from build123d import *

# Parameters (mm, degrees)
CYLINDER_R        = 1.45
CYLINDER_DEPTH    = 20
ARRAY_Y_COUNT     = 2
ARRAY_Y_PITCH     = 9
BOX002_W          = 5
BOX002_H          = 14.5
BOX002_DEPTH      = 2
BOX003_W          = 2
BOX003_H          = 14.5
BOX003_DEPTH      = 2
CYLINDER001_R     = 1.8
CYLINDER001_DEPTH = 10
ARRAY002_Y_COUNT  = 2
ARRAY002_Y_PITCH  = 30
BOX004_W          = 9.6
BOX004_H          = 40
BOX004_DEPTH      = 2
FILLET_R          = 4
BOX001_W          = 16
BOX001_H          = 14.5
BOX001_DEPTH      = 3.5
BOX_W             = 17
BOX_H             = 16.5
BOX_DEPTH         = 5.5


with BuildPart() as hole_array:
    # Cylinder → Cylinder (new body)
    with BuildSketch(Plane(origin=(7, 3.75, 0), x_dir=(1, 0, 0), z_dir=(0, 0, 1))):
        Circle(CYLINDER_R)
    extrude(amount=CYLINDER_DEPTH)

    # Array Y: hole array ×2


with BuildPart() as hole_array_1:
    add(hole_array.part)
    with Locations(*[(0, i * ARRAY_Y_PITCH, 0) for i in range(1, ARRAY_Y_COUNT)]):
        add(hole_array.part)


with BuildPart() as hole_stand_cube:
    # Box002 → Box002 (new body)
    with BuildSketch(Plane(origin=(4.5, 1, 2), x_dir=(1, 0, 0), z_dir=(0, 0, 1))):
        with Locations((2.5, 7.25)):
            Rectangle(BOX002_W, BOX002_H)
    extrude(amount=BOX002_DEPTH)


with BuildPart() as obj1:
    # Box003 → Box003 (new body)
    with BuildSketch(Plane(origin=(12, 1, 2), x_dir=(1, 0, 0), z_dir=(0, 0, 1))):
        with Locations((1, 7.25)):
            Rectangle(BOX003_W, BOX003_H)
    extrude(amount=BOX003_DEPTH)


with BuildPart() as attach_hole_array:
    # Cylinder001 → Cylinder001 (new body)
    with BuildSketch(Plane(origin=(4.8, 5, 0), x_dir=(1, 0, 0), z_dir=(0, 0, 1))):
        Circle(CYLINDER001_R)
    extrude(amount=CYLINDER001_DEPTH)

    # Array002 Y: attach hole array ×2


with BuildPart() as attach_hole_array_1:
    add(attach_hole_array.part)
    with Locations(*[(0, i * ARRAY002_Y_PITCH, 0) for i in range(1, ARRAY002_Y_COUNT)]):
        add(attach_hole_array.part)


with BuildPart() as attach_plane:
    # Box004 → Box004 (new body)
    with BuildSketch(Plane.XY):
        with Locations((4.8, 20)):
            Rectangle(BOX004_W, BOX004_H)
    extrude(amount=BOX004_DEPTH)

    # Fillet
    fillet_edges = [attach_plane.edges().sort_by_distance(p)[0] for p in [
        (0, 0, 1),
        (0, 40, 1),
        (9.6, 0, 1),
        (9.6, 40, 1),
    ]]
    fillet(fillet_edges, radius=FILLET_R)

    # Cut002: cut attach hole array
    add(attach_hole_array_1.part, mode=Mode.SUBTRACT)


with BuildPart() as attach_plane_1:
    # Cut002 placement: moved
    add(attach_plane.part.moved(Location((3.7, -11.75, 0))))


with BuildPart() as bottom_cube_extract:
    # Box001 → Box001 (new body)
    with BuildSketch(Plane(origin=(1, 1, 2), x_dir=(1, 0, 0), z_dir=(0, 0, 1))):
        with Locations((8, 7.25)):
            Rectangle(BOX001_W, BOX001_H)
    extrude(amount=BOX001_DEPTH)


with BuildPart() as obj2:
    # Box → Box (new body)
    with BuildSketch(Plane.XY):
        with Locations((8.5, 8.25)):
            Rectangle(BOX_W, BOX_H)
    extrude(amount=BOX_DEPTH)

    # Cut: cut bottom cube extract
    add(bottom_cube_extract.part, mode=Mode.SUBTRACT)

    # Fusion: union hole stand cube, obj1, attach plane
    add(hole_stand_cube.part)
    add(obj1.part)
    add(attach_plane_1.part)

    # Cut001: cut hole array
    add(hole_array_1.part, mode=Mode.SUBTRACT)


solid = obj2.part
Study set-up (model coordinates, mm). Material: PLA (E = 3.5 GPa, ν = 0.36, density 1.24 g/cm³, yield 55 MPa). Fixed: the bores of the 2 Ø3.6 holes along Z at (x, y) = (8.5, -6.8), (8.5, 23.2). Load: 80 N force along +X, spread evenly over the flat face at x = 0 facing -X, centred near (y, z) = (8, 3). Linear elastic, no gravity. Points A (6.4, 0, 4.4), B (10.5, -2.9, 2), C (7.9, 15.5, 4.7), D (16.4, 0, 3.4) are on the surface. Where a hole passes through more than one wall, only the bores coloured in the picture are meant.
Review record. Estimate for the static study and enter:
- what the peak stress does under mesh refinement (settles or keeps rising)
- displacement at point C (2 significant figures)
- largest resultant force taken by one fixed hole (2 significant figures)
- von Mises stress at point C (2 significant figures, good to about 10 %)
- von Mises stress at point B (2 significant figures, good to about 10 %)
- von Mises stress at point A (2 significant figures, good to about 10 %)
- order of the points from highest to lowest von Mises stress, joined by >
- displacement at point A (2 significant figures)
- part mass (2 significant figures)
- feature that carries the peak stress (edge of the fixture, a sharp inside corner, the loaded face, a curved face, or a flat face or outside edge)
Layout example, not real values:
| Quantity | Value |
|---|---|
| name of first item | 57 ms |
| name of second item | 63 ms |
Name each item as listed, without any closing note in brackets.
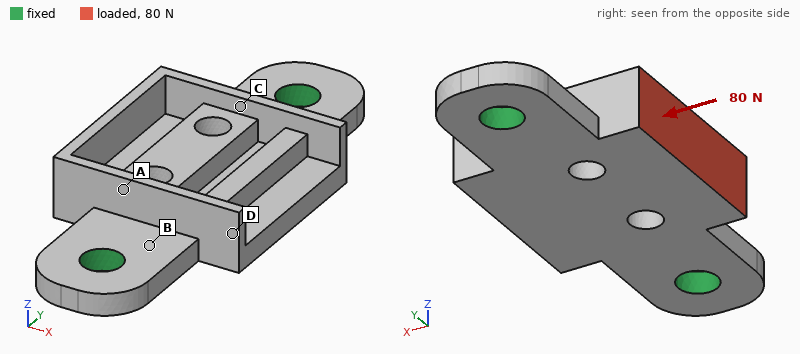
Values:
| Quantity | Value |
|---|---|
| what the peak stress does under mesh refinement | keeps rising |
| displacement at point C | 0.060 mm |
| largest resultant force taken by one fixed hole | 40 N |
| von Mises stress at point C | 2.9 MPa |
| von Mises stress at point B | 11 MPa |
| von Mises stress at point A | 5.5 MPa |
| order of the points from highest to lowest von Mises stress, joined by > | B > A > C > D |
| displacement at point A | 0.063 mm |
| part mass | 1.6 g |
| feature that carries the peak stress | edge of the fixture |
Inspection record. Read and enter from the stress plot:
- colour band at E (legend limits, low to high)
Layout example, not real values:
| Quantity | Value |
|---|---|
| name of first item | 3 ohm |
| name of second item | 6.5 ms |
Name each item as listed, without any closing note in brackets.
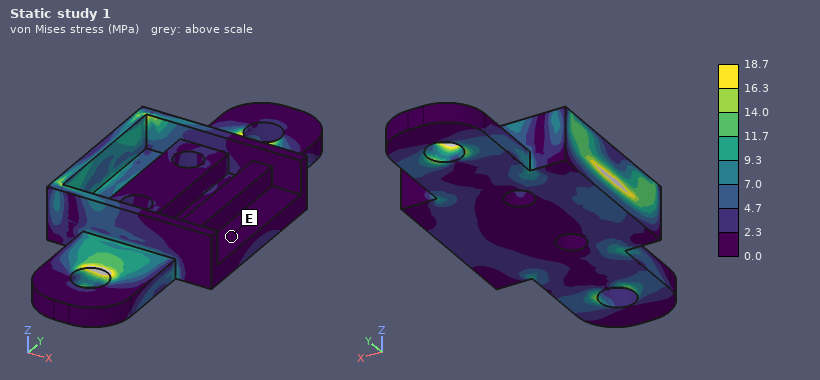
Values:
| Quantity | Value |
|---|---|
| colour band at E | 0.0 to 2.3 MPa |
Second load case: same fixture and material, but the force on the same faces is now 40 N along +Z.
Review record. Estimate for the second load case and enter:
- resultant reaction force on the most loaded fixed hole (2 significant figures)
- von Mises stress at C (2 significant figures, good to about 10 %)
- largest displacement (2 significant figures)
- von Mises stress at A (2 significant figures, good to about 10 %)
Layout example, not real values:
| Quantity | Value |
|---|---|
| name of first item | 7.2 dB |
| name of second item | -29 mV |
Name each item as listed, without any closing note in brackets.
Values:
| Quantity | Value |
|---|---|
| resultant reaction force on the most loaded fixed hole | 26 N |
| von Mises stress at C | 6.7 MPa |
| largest displacement | 0.36 mm |
| von Mises stress at A | 6.4 MPa |
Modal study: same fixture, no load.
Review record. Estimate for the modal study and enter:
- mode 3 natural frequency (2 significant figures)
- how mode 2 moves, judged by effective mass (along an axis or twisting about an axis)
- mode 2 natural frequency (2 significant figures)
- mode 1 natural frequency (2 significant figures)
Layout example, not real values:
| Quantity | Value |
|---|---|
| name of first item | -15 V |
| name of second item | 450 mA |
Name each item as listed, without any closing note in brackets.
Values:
| Quantity | Value |
|---|---|
| mode 3 natural frequency | 9000 Hz |
| how mode 2 moves, judged by effective mass | along Z |
| mode 2 natural frequency | 4300 Hz |
| mode 1 natural frequency | 3200 Hz |
